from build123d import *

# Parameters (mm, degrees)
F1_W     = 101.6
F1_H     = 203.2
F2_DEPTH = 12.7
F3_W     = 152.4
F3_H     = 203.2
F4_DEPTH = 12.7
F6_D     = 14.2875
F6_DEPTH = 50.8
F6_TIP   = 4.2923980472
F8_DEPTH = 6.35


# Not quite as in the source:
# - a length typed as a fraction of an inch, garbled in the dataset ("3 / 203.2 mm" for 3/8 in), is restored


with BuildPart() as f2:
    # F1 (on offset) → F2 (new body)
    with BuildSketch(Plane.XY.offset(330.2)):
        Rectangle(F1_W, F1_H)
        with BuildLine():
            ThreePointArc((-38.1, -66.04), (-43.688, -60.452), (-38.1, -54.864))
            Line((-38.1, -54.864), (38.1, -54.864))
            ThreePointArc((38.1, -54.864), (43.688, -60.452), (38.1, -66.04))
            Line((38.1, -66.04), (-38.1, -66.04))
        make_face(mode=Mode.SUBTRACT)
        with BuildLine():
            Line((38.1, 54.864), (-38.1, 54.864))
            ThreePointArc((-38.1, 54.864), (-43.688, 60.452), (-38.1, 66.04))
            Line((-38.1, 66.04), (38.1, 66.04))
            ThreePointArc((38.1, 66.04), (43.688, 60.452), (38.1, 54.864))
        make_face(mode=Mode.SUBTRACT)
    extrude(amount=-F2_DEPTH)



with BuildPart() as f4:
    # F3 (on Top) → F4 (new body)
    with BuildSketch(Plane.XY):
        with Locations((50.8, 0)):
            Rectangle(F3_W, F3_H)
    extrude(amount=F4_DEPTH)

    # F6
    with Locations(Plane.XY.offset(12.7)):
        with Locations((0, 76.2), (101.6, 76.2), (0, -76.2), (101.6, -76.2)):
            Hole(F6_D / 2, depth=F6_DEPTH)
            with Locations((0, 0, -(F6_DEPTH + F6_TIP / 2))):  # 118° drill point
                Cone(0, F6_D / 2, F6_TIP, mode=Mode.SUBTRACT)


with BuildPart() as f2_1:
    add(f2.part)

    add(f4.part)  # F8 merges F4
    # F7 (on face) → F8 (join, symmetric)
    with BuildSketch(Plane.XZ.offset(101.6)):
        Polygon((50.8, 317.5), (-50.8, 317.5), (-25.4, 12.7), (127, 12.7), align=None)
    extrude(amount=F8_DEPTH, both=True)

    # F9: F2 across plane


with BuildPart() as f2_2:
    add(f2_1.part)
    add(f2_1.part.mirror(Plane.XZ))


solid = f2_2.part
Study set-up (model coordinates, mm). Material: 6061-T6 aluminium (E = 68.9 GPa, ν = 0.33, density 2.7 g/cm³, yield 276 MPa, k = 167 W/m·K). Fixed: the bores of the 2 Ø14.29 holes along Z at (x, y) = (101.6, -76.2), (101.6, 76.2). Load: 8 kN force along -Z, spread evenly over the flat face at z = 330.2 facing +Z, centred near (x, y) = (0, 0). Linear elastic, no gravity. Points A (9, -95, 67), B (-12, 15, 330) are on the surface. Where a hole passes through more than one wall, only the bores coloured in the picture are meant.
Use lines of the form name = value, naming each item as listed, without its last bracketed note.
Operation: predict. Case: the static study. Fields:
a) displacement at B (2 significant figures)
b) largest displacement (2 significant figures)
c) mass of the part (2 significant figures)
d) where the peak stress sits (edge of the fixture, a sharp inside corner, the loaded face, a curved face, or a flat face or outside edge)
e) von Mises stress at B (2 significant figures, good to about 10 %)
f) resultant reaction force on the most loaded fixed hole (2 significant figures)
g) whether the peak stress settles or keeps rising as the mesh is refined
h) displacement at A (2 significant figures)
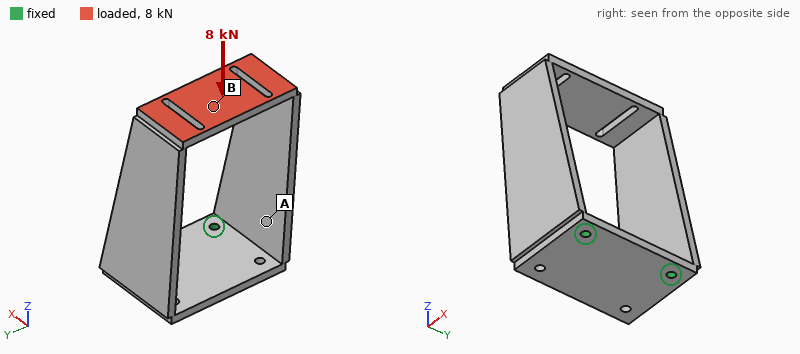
displacement at B = 2.4 mm
largest displacement = 2.6 mm
mass of the part = 4.3 kg
where the peak stress sits = edge of the fixture
von Mises stress at B = 33 MPa
resultant reaction force on the most loaded fixed hole = 4.0 kN
whether the peak stress settles or keeps rising as the mesh is refined = keeps rising
displacement at A = 0.72 mm
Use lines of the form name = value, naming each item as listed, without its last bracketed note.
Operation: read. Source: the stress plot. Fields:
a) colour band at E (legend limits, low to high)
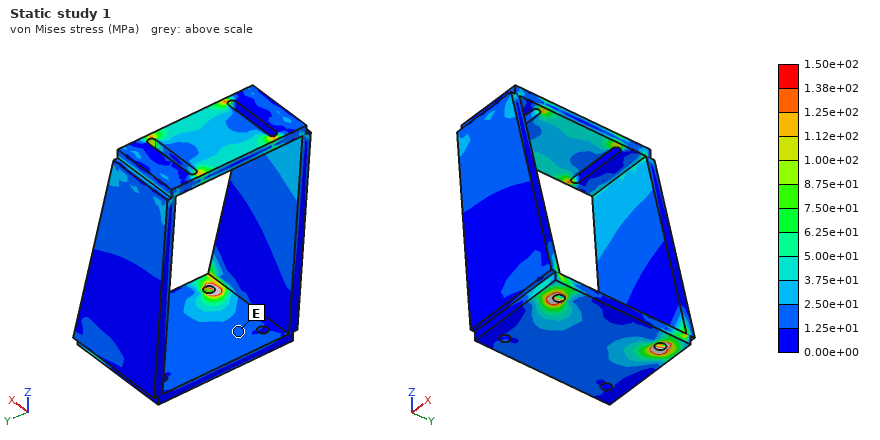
colour band at E = 1.25e+01 to 2.50e+01 MPa
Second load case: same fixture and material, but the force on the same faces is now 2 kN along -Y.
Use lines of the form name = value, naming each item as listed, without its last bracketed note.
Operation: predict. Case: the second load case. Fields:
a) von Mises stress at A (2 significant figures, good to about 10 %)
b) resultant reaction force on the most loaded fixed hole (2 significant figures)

von Mises stress at A = 33 MPa
resultant reaction force on the most loaded fixed hole = 3.0 kN
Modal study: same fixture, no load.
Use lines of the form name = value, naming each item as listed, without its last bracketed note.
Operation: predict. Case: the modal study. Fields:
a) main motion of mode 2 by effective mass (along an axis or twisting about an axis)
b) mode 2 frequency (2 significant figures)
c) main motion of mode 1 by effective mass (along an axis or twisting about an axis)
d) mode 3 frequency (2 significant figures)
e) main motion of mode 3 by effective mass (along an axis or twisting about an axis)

main motion of mode 2 by effective mass = along X
mode 2 frequency = 140 Hz
main motion of mode 1 by effective mass = along Y
mode 3 frequency = 260 Hz
main motion of mode 3 by effective mass = twisting about Z
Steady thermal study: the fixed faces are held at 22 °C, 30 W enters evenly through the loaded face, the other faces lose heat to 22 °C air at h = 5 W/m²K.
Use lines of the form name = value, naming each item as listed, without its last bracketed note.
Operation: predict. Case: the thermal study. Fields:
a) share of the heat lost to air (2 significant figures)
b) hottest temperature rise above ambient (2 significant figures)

share of the heat lost to air = 36 %
hottest temperature rise above ambient = 25 K
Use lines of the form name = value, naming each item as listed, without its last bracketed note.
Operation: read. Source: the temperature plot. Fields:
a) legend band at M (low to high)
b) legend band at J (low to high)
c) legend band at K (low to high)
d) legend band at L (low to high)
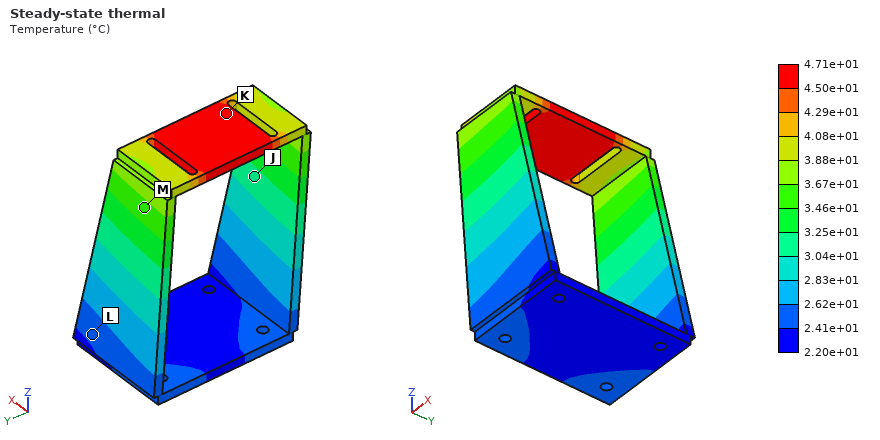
legend band at M = 3.46e+01 to 3.67e+01 °C
legend band at J = 3.04e+01 to 3.25e+01 °C
legend band at K = 4.50e+01 to 4.71e+01 °C
legend band at L = 2.41e+01 to 2.62e+01 °C
